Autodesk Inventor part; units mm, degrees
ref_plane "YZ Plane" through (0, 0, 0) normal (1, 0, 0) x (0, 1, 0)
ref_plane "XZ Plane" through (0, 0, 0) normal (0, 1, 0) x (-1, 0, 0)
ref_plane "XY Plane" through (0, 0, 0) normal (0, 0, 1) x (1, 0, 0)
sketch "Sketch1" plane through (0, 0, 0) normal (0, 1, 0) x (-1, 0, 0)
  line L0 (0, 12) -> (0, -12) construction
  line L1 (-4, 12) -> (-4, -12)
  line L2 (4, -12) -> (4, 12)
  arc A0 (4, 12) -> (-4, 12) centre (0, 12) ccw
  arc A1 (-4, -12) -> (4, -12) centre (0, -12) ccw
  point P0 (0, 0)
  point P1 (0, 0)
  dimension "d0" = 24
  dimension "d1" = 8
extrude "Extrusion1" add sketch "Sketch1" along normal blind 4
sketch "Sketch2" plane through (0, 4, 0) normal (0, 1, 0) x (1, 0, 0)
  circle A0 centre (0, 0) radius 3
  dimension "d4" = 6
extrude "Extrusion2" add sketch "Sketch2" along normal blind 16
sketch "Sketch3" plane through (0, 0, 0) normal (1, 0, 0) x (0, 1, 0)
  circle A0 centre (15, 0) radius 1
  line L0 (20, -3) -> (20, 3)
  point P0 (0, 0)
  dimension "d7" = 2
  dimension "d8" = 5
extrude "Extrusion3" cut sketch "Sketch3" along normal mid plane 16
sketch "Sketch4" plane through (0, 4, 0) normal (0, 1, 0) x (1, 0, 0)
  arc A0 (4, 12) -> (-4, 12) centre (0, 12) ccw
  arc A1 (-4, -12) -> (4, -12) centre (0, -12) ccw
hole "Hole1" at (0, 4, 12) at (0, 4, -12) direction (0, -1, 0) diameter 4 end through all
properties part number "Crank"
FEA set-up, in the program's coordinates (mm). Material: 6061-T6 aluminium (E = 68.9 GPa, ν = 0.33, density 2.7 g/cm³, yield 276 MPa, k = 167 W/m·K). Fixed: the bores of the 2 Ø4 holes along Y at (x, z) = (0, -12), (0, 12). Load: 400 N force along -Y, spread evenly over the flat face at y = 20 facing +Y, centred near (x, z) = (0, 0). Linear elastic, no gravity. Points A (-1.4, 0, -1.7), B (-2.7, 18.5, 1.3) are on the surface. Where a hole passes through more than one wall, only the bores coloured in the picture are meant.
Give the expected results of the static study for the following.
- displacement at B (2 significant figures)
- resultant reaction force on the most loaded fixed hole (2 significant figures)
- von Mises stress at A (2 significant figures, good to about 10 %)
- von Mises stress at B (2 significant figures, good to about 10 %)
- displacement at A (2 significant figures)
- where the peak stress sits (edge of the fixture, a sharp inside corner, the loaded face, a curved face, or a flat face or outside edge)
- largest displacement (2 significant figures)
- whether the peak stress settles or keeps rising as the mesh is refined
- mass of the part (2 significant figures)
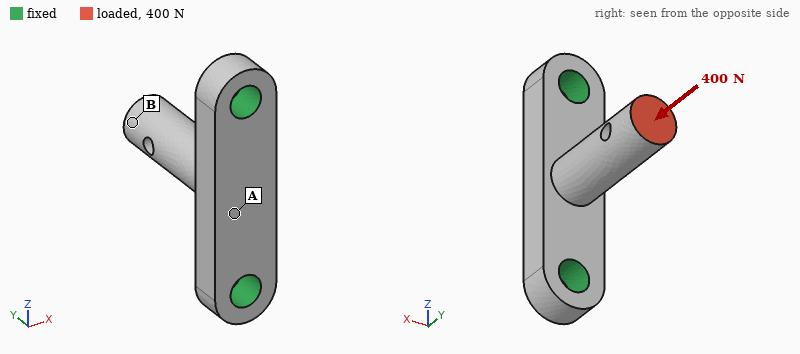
11 µm
200 N
28 MPa
14 MPa
7.2 µm
edge of the fixture
11 µm
keeps rising
3.5 g
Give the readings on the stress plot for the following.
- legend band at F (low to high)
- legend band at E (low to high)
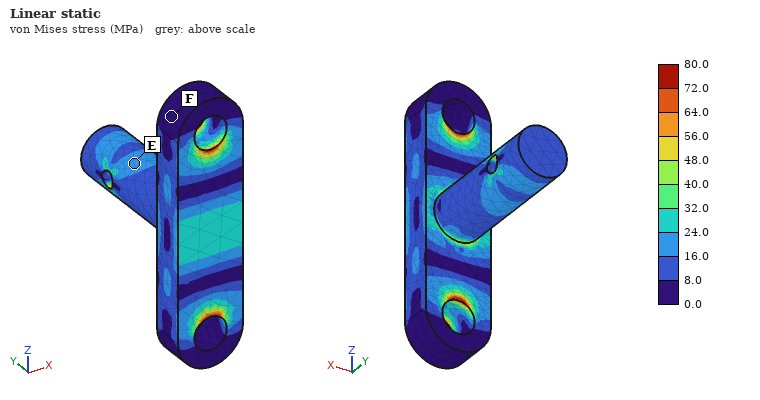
0.0 to 8.0 MPa
16.0 to 24.0 MPa
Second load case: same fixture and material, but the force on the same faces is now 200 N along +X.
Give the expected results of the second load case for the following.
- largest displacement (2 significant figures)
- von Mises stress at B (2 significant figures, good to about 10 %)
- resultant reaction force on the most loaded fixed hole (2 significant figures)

0.18 mm
15 MPa
100 N
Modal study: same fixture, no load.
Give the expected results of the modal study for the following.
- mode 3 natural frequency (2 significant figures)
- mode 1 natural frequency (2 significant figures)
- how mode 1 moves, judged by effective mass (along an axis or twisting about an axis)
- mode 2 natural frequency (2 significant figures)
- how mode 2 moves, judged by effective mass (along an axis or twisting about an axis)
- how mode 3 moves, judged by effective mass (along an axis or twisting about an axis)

25 kHz
8800 Hz
along X
12 kHz
along Z
along Y
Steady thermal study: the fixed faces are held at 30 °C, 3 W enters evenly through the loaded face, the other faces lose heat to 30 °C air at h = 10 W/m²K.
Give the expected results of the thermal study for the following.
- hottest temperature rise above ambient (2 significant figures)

14 K
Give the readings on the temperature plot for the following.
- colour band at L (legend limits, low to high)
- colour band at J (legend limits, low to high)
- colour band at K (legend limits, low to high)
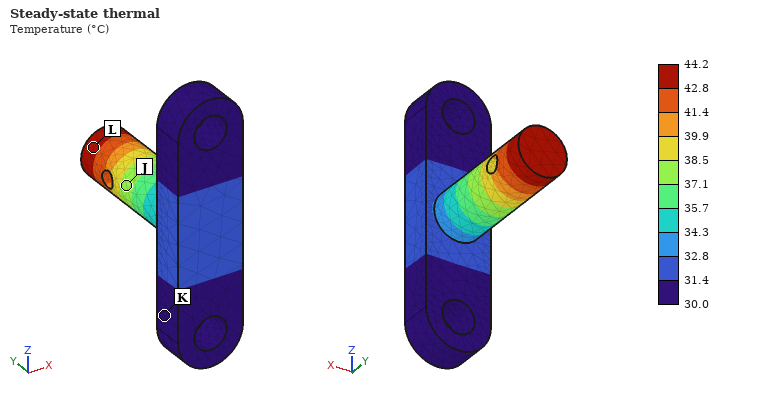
42.8 to 44.2 °C
37.1 to 38.5 °C
30.0 to 31.4 °C
